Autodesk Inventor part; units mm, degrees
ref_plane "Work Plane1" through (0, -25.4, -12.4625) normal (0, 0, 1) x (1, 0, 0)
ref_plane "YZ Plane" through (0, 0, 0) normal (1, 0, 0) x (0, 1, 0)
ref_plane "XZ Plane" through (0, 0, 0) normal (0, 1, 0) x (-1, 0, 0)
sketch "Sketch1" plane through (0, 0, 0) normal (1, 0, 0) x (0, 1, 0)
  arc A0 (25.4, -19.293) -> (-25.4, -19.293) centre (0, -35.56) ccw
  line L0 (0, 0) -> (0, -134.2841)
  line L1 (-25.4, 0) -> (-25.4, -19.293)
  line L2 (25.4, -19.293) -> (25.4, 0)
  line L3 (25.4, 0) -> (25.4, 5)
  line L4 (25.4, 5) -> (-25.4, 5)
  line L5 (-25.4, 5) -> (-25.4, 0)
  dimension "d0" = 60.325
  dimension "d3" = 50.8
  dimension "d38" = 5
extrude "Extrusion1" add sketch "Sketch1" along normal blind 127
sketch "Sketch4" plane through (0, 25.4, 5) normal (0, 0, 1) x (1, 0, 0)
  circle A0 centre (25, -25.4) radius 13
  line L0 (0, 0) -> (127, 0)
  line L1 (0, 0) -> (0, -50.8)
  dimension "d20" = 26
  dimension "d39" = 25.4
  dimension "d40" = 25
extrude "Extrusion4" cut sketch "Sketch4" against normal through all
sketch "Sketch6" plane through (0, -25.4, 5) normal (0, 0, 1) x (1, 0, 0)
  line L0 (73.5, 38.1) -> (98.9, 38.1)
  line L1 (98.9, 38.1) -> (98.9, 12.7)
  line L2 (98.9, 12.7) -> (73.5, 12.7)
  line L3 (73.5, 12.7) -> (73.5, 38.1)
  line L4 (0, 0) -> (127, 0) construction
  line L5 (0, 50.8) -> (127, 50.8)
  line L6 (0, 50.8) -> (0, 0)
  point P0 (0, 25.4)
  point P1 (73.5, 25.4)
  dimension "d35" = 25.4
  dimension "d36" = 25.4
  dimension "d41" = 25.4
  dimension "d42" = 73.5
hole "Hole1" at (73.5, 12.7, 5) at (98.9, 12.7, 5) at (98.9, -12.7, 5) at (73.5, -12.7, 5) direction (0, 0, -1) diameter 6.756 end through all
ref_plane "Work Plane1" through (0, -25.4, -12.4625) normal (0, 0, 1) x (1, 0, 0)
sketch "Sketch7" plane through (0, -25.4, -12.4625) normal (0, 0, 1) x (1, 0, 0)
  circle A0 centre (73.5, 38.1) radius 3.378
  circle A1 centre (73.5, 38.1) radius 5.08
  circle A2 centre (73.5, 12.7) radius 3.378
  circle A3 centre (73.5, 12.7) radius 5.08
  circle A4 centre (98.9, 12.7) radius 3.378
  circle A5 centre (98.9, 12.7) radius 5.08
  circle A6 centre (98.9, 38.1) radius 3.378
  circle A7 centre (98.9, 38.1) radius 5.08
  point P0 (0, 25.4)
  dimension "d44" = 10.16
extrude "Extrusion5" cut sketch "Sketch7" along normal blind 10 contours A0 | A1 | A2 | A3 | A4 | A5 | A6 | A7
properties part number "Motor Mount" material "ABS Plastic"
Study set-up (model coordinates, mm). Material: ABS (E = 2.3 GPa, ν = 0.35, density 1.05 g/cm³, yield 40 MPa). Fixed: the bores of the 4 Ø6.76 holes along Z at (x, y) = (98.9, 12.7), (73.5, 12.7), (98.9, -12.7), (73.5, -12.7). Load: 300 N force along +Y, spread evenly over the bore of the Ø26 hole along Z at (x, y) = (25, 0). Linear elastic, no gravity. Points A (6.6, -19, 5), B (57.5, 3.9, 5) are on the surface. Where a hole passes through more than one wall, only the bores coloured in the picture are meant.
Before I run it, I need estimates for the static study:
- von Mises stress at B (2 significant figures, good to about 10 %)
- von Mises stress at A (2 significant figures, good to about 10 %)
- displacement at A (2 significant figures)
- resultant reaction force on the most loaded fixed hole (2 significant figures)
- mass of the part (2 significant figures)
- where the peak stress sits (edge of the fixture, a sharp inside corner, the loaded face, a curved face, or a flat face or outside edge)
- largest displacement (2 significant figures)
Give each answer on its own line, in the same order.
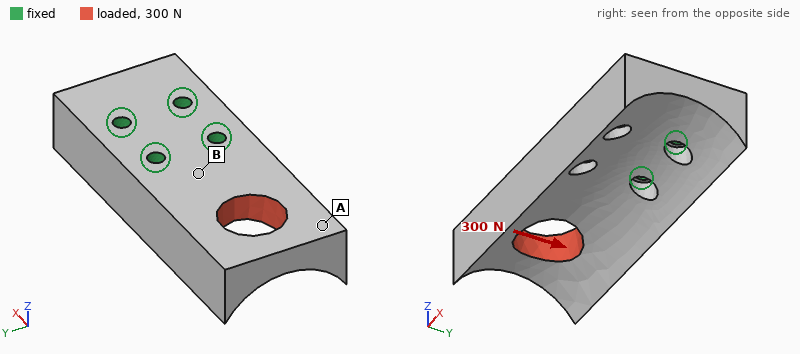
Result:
1.7 MPa
0.65 MPa
0.14 mm
360 N
89 g
edge of the fixture
0.16 mm
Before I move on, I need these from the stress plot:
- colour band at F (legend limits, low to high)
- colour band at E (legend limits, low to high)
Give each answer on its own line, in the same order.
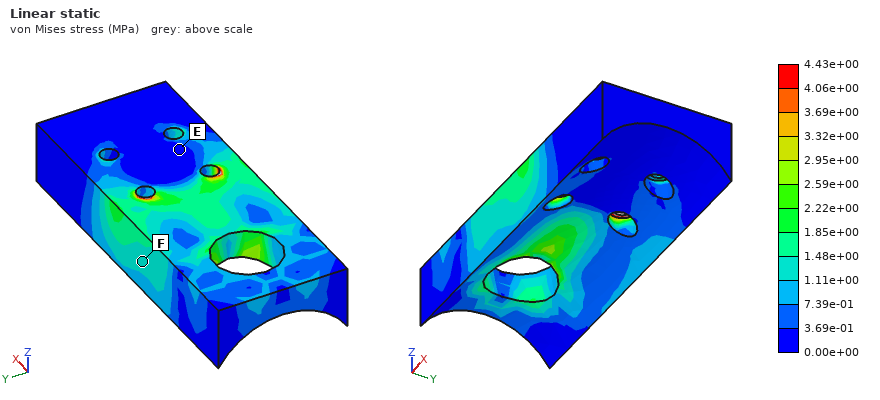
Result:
1.11e+00 to 1.48e+00 MPa
0.00e+00 to 3.69e-01 MPa
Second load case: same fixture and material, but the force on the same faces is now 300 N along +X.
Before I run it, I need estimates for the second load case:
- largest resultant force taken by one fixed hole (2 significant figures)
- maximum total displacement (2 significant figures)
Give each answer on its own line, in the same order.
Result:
120 N
34 µm
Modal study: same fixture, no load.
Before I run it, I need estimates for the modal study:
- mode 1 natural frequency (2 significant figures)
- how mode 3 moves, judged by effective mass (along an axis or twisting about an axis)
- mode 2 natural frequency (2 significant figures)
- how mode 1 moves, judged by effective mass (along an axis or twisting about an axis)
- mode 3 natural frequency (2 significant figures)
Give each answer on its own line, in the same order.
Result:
660 Hz
along Y
1200 Hz
along Z
1500 Hz
